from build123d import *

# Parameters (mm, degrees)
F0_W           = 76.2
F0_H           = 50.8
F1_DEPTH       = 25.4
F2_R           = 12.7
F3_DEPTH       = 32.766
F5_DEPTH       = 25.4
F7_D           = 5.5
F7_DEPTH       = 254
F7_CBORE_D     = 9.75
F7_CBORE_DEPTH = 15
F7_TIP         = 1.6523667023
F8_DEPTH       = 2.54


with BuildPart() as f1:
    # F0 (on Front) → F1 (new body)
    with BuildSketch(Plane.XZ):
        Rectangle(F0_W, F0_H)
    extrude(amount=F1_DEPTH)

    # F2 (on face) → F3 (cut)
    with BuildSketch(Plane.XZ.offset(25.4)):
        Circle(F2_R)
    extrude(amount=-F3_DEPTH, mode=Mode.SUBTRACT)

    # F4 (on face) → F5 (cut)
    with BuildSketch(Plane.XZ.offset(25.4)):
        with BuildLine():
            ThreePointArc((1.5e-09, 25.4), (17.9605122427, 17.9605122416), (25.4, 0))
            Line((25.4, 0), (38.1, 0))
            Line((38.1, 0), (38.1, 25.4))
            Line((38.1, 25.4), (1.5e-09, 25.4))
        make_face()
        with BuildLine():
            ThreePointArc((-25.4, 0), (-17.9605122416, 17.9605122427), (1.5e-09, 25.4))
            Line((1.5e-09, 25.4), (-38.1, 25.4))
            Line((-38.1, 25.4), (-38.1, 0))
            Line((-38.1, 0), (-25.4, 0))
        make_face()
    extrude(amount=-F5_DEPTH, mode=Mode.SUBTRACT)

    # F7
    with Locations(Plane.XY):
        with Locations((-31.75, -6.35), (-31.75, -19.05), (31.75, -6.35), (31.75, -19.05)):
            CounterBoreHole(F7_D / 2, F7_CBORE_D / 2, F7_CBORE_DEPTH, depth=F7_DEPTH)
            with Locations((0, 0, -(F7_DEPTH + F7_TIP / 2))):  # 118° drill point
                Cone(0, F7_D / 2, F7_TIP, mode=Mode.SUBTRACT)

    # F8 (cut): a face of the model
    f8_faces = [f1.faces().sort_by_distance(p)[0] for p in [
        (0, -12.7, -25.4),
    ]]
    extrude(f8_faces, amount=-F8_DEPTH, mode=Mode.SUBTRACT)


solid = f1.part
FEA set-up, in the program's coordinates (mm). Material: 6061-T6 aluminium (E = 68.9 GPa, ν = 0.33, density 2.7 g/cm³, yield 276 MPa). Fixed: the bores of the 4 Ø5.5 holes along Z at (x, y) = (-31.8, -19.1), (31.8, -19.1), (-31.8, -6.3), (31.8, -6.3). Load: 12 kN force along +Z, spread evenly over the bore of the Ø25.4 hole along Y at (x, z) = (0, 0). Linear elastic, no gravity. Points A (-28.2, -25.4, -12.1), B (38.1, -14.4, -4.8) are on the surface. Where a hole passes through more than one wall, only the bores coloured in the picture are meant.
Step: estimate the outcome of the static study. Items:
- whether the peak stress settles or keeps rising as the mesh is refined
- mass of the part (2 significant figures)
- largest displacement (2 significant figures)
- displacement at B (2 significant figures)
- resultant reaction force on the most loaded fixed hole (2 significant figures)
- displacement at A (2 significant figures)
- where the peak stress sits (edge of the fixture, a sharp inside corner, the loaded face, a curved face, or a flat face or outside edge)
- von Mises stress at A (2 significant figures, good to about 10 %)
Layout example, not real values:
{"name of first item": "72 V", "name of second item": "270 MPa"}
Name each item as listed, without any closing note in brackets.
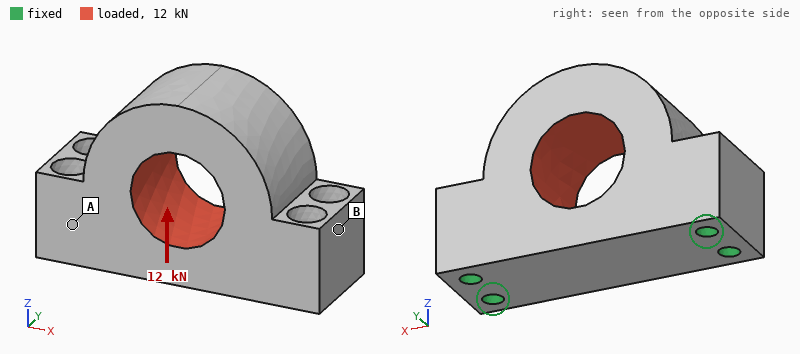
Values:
{"whether the peak stress settles or keeps rising as the mesh is refined": "keeps rising", "mass of the part": "140 g", "largest displacement": "24 µm", "displacement at B": "5.2 µm", "resultant reaction force on the most loaded fixed hole": "3.3 kN", "displacement at A": "6.6 µm", "where the peak stress sits": "edge of the fixture", "von Mises stress at A": "30 MPa"}
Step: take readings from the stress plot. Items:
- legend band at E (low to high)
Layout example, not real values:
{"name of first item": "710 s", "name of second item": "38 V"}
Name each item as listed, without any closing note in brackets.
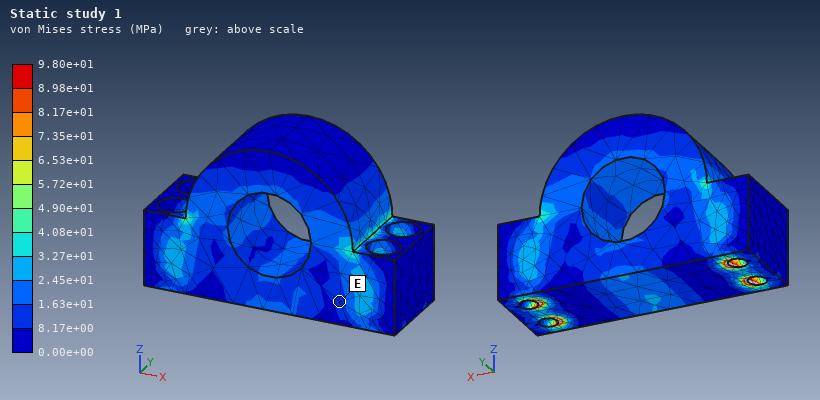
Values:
{"legend band at E": "8.17e+00 to 1.63e+01 MPa"}
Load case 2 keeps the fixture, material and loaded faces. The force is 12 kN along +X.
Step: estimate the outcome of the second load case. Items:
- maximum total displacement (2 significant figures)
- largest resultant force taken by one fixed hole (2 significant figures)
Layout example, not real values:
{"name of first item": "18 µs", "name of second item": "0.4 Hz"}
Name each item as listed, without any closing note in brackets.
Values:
{"maximum total displacement": "25 µm", "largest resultant force taken by one fixed hole": "3.5 kN"}
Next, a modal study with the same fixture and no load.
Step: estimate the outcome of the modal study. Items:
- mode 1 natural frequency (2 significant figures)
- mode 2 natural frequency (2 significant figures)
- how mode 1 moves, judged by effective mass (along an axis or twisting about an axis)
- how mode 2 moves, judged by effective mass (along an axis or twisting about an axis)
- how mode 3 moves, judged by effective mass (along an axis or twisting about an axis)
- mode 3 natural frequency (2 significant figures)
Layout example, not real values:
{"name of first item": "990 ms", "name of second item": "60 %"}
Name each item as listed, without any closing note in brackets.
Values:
{"mode 1 natural frequency": "5600 Hz", "mode 2 natural frequency": "12 kHz", "how mode 1 moves, judged by effective mass": "along Y", "how mode 2 moves, judged by effective mass": "along X", "how mode 3 moves, judged by effective mass": "along Z", "mode 3 natural frequency": "13 kHz"}
